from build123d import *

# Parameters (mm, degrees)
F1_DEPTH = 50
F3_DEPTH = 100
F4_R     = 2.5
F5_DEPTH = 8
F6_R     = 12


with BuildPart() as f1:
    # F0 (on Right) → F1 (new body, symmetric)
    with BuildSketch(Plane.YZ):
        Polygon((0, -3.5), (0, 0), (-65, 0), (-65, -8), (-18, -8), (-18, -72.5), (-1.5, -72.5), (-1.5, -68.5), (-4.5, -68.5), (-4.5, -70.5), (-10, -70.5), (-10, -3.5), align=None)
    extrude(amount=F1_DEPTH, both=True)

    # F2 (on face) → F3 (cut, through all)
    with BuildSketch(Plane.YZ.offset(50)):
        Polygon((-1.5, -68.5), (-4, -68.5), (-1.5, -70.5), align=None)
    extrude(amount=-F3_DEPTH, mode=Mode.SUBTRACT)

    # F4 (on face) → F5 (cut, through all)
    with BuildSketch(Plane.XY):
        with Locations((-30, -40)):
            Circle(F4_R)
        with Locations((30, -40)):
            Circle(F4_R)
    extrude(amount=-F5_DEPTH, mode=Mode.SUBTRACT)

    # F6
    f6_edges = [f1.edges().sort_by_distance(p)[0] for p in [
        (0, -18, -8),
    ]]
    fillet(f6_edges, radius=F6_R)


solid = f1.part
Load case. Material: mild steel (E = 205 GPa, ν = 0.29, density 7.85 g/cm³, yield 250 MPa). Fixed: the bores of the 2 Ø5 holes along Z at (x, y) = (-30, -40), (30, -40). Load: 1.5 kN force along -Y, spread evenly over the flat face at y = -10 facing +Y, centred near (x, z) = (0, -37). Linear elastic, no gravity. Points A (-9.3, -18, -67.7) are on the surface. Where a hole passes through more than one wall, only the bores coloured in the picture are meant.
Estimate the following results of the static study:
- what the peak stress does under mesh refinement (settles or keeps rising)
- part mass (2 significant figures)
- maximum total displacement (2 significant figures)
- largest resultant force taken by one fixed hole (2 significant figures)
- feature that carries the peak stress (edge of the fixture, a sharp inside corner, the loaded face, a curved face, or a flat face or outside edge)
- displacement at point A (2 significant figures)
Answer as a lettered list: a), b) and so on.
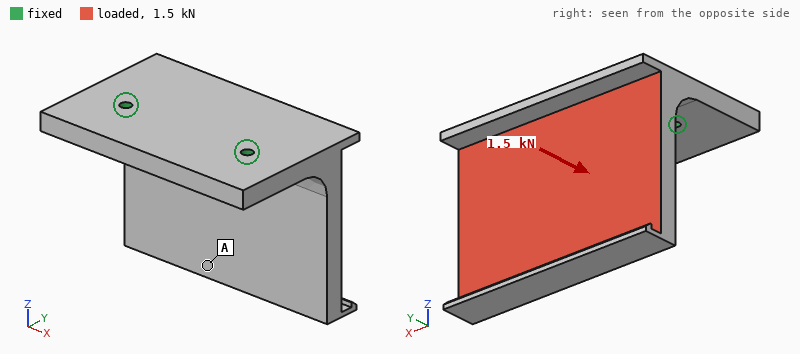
a) keeps rising
b) 820 g
c) 0.14 mm
d) 760 N
e) edge of the fixture
f) 0.12 mm
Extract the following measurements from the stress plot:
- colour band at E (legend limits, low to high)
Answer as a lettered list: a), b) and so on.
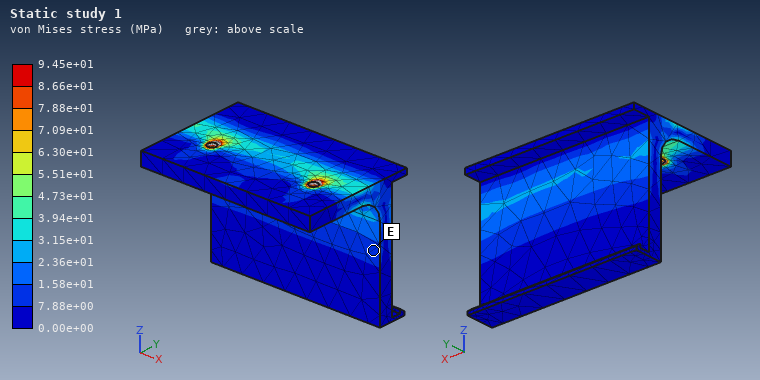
a) 7.88e+00 to 1.58e+01 MPa
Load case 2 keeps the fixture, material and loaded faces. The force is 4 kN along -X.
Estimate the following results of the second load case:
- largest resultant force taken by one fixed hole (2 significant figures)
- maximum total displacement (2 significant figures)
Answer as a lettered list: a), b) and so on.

a) 3.4 kN
b) 45 µm
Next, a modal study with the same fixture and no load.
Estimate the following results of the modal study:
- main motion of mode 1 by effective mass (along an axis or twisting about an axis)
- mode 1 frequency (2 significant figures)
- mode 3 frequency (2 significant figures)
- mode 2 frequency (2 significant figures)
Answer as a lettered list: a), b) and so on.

a) along Y
b) 880 Hz
c) 3000 Hz
d) 1900 Hz
